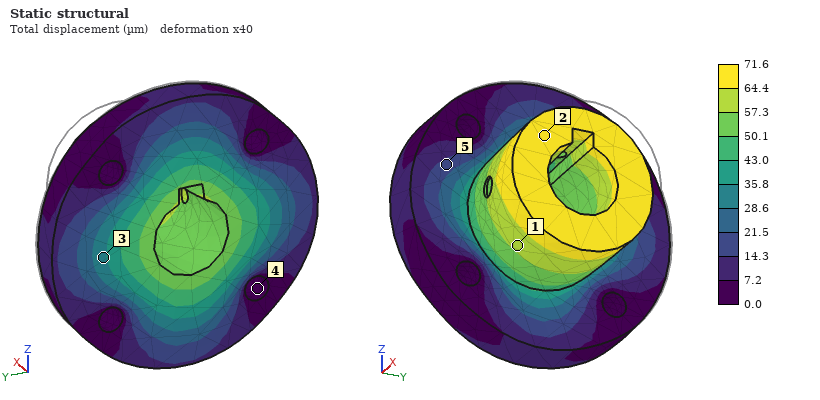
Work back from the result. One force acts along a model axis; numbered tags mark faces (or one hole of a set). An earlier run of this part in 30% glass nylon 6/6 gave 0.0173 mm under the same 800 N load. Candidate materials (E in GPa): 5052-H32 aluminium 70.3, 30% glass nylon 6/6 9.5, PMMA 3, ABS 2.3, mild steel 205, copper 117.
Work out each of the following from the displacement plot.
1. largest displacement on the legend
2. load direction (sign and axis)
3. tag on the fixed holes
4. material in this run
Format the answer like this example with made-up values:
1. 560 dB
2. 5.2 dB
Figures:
1. 71.6 µm
2. -X
3. 4
4. ABS
